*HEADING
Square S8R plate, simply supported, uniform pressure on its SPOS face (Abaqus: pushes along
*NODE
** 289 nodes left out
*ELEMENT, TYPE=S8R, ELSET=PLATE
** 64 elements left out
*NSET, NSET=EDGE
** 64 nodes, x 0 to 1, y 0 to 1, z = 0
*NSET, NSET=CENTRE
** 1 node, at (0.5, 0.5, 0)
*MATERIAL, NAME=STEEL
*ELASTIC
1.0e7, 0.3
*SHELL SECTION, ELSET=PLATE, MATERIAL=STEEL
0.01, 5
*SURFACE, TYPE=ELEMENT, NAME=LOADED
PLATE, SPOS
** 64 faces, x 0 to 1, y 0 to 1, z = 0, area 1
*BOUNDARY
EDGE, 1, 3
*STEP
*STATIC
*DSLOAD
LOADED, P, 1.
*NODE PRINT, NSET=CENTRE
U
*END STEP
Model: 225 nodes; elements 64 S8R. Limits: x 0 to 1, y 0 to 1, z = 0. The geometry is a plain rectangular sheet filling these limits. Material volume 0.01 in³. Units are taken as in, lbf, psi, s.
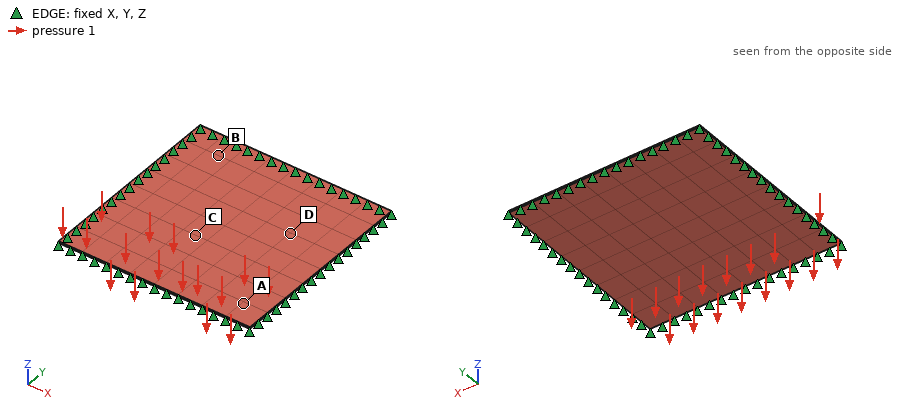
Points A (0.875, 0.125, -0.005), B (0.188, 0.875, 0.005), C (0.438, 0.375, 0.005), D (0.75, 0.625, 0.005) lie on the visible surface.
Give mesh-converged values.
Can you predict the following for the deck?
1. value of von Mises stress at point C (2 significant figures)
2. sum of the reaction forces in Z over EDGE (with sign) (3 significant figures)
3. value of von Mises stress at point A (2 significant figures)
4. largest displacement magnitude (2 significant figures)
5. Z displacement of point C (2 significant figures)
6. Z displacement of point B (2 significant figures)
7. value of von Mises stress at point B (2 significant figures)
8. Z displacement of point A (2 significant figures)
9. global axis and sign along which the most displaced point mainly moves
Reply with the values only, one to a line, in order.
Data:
2700 psi
1.00 lbf
2800 psi
0.0045 in
-0.0041 in
-0.0010 in
2600 psi
-7.3e-04 in
-Z
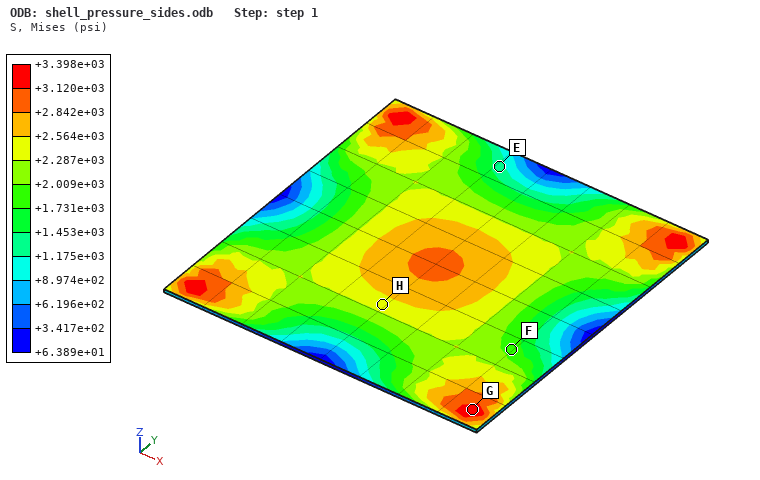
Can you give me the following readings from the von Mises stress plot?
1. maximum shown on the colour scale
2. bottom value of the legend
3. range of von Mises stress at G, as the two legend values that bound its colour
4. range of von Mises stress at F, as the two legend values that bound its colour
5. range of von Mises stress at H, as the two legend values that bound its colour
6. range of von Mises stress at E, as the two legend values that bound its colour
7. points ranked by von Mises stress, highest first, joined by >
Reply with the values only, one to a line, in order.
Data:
+3.398e+03 psi
+6.389e+01 psi
+3.120e+03 to +3.398e+03 psi
+1.731e+03 to +2.009e+03 psi
+2.287e+03 to +2.564e+03 psi
+1.175e+03 to +1.453e+03 psi
G > H > F > E
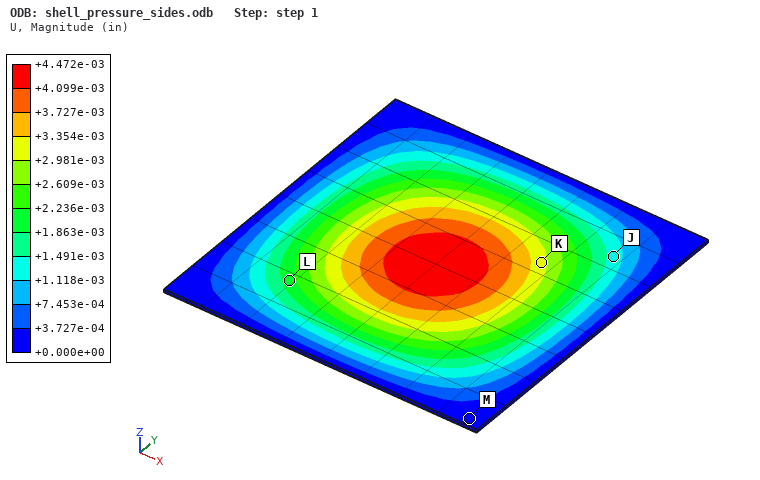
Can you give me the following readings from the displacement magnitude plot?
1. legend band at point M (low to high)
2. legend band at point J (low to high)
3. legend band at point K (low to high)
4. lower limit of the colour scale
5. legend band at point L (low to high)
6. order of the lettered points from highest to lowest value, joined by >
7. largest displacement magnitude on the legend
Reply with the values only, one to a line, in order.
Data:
+0.000e+00 to +3.727e-04 in
+1.118e-03 to +1.491e-03 in
+2.981e-03 to +3.354e-03 in
+0.000e+00 in
+1.863e-03 to +2.236e-03 in
K > L > J > M
+4.472e-03 in
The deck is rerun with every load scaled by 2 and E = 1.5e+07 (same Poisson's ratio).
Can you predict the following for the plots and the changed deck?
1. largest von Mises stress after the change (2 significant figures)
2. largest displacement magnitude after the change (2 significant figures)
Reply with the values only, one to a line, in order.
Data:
6800 psi
0.0060 in
